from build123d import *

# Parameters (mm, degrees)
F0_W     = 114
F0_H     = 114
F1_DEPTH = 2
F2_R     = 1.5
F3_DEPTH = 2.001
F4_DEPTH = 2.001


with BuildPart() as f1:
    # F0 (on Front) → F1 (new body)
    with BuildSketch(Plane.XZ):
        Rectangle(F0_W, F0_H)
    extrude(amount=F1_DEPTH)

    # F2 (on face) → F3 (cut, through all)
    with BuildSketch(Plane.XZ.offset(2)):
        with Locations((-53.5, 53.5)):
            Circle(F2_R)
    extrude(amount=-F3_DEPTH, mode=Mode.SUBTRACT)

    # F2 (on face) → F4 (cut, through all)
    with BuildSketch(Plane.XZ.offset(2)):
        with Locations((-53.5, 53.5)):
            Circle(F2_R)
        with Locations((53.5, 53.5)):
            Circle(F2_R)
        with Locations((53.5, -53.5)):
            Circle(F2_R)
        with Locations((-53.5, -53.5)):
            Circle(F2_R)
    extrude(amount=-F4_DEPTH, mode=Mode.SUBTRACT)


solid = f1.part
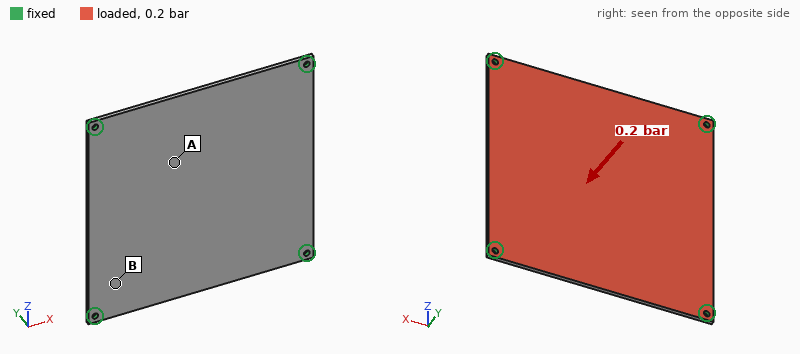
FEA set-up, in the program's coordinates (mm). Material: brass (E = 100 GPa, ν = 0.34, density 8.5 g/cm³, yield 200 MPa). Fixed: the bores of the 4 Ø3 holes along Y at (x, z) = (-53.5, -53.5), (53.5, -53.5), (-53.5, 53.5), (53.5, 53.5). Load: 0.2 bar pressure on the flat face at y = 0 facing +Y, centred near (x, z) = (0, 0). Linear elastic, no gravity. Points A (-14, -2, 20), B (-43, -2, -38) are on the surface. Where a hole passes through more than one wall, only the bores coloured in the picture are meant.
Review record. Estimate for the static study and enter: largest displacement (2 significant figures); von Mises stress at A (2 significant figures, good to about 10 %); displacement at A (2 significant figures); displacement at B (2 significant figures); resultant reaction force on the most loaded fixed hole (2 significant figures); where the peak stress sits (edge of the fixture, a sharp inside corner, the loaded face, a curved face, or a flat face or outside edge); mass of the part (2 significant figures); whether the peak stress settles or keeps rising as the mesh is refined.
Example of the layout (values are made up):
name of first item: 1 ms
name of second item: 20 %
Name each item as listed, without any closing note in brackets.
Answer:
largest displacement: 0.34 mm
von Mises stress at A: 19 MPa
displacement at A: 0.29 mm
displacement at B: 0.097 mm
resultant reaction force on the most loaded fixed hole: 65 N
where the peak stress sits: edge of the fixture
mass of the part: 220 g
whether the peak stress settles or keeps rising as the mesh is refined: keeps rising
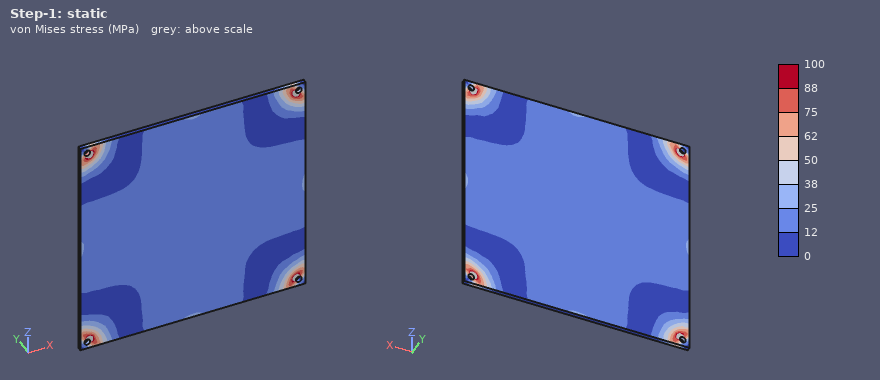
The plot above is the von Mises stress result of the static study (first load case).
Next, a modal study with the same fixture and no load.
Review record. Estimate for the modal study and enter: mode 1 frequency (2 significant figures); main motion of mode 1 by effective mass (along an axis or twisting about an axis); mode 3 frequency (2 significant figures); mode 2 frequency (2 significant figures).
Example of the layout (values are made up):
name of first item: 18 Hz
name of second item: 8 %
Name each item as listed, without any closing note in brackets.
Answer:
mode 1 frequency: 360 Hz
main motion of mode 1 by effective mass: along Y
mode 3 frequency: 650 Hz
mode 2 frequency: 650 Hz
